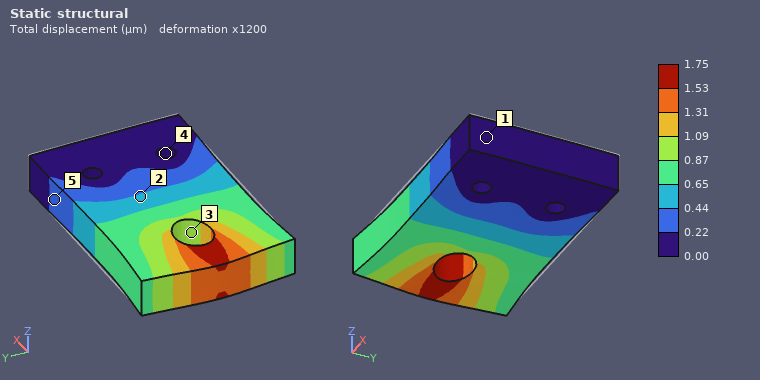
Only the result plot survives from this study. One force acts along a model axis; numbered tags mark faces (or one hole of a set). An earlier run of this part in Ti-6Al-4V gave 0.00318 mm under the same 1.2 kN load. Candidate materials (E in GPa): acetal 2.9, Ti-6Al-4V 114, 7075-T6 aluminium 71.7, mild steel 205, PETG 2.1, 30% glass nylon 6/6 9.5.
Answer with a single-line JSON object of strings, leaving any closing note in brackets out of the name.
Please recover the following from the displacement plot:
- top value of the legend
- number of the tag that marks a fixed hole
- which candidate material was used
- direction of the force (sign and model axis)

{"top value of the legend": "1.75 µm", "number of the tag that marks a fixed hole": "4", "which candidate material was used": "mild steel", "direction of the force": "-X"}
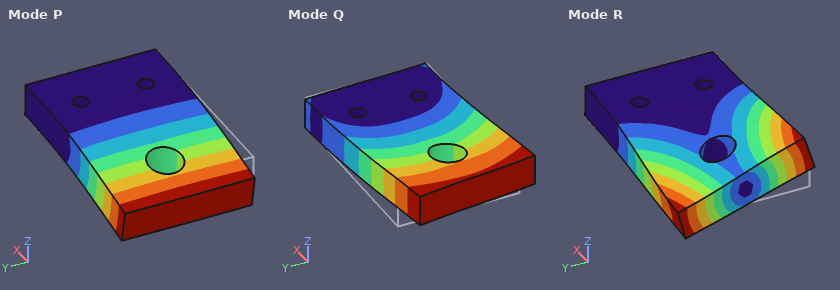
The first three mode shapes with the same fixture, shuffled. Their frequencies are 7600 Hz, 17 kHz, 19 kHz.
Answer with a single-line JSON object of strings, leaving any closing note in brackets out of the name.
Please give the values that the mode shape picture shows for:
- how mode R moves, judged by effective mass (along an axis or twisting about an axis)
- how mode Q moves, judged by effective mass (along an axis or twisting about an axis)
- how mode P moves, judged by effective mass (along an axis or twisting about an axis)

{"how mode R moves, judged by effective mass": "twisting about X", "how mode Q moves, judged by effective mass": "along Y", "how mode P moves, judged by effective mass": "along Z"}
